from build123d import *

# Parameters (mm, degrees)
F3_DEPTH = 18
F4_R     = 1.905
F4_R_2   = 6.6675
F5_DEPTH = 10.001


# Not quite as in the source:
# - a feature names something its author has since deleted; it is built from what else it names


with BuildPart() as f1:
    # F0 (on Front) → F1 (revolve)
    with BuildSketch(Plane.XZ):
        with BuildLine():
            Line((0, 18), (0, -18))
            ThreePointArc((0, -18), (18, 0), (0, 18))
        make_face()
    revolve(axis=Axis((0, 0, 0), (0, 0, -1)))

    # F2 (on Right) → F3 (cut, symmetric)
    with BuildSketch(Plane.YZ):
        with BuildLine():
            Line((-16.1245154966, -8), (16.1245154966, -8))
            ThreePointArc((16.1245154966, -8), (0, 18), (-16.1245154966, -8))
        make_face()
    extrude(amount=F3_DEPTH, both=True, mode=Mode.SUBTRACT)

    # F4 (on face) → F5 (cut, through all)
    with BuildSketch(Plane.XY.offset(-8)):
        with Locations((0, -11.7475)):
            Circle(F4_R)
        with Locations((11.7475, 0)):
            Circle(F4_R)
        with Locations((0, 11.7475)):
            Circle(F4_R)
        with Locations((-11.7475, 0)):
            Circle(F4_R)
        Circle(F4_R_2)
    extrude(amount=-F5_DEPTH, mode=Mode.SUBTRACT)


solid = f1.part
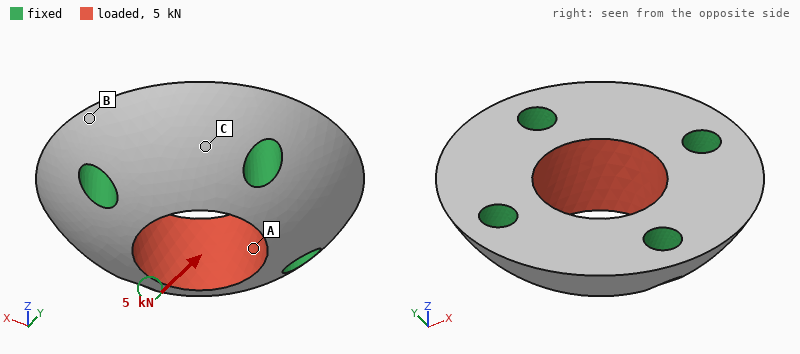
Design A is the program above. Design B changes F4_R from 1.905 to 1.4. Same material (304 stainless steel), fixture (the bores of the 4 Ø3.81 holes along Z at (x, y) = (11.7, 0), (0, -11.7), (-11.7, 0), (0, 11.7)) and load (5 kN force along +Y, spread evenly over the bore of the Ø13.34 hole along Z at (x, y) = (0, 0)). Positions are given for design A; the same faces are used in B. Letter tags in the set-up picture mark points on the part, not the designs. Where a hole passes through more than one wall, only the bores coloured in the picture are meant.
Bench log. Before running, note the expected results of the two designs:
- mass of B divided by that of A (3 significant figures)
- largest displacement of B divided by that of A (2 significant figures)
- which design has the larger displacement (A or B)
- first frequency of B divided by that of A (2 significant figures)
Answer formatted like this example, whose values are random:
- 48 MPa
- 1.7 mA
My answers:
- 1.04
- 1.1
- B
- 0.87
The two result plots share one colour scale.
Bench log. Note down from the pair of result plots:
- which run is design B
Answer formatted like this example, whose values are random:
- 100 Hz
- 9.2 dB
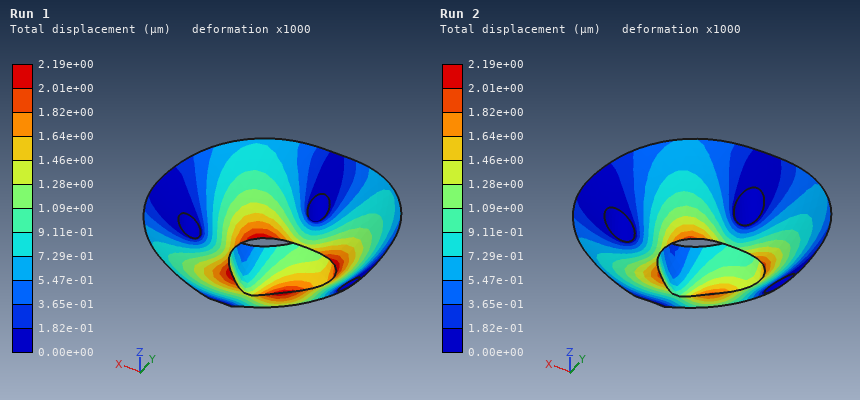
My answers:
- Run 1
